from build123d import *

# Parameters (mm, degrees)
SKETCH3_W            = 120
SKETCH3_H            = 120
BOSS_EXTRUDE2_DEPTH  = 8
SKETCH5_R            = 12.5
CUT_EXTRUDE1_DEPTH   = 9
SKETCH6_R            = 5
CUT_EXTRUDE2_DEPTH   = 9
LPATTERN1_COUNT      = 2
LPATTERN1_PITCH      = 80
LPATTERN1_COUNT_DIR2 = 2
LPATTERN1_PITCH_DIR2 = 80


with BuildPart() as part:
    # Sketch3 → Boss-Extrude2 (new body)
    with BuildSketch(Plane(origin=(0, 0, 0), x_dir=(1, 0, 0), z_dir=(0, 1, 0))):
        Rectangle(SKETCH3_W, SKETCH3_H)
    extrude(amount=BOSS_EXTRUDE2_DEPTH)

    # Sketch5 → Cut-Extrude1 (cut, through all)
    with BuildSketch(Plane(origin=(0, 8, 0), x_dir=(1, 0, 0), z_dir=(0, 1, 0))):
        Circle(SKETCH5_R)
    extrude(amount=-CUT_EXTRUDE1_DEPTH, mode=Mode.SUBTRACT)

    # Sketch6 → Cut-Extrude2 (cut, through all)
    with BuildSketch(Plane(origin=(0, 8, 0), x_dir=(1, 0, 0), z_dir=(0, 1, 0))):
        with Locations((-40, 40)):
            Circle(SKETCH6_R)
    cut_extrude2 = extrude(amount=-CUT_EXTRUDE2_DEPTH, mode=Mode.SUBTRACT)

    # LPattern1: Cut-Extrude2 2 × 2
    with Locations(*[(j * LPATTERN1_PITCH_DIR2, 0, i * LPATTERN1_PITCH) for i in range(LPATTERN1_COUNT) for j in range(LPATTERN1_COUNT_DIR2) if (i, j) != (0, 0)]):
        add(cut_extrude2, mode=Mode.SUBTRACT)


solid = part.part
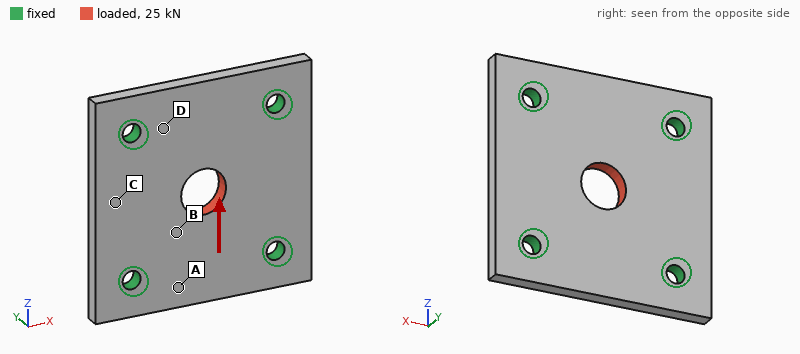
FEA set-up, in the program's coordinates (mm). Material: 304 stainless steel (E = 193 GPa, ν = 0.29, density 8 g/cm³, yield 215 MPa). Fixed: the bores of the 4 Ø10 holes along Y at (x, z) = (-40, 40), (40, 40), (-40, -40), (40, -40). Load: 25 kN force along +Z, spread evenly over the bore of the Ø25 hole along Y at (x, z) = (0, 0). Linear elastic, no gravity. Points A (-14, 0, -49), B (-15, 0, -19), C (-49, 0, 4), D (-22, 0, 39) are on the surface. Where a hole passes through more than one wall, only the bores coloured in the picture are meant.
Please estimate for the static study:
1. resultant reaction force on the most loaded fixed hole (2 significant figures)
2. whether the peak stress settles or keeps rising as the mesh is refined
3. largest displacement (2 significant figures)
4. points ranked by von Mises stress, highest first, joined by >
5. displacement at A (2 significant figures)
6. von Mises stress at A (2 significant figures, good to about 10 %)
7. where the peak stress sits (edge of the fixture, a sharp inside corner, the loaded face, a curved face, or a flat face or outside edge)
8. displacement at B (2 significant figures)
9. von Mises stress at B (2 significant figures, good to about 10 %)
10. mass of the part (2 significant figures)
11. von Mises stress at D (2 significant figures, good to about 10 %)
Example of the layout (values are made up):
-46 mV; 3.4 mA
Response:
6.7 kN; keeps rising; 9.4 µm; B > D > A > C; 4.9 µm; 13 MPa; edge of the fixture; 6.1 µm; 31 MPa; 870 g; 22 MPa
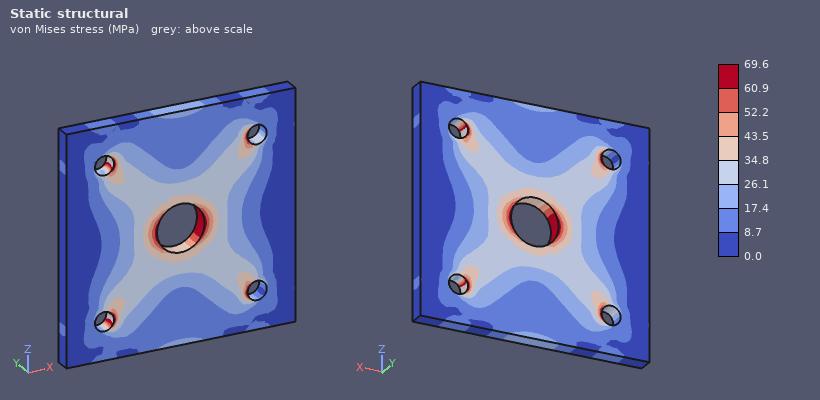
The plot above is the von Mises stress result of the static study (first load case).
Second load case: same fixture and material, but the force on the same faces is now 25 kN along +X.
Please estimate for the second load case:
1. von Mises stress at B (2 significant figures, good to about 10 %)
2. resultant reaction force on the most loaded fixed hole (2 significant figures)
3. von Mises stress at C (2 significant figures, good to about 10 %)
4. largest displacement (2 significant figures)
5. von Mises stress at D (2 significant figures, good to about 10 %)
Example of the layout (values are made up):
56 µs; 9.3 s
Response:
30 MPa; 6.7 kN; 10 MPa; 9.4 µm; 20 MPa
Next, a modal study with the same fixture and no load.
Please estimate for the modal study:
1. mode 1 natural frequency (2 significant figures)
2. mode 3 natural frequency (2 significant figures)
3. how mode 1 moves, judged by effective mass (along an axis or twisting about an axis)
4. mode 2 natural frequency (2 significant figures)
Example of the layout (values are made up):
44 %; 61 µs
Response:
4800 Hz; 6500 Hz; along Y; 6400 Hz
